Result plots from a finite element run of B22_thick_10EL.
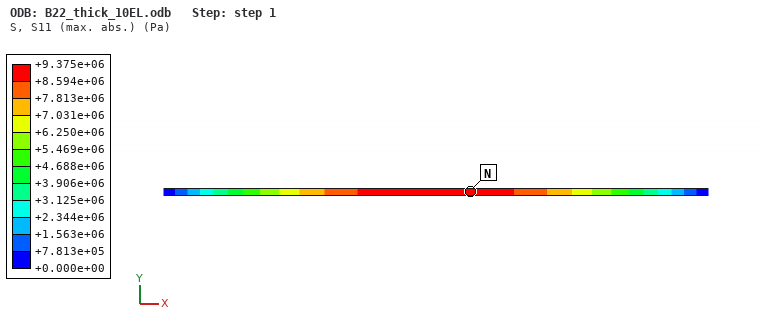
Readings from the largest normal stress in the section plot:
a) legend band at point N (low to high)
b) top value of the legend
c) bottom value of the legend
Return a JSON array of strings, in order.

["+8.594e+06 to +9.375e+06 Pa", "+9.375e+06 Pa", "+0.000e+00 Pa"]
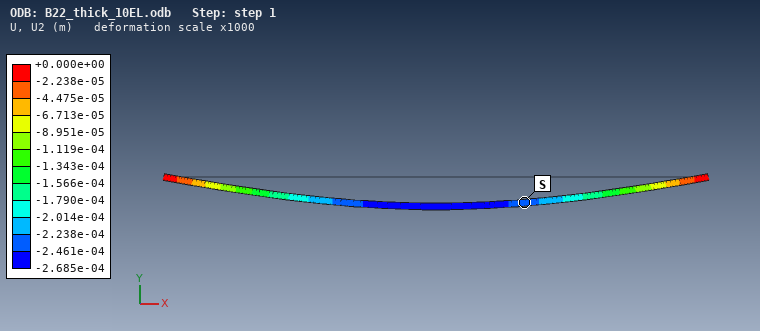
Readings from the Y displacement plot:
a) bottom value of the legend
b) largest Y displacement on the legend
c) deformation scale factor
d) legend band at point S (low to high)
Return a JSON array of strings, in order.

["-2.685e-04 m", "+0.000e+00 m", "1000", "-2.461e-04 to -2.238e-04 m"]
